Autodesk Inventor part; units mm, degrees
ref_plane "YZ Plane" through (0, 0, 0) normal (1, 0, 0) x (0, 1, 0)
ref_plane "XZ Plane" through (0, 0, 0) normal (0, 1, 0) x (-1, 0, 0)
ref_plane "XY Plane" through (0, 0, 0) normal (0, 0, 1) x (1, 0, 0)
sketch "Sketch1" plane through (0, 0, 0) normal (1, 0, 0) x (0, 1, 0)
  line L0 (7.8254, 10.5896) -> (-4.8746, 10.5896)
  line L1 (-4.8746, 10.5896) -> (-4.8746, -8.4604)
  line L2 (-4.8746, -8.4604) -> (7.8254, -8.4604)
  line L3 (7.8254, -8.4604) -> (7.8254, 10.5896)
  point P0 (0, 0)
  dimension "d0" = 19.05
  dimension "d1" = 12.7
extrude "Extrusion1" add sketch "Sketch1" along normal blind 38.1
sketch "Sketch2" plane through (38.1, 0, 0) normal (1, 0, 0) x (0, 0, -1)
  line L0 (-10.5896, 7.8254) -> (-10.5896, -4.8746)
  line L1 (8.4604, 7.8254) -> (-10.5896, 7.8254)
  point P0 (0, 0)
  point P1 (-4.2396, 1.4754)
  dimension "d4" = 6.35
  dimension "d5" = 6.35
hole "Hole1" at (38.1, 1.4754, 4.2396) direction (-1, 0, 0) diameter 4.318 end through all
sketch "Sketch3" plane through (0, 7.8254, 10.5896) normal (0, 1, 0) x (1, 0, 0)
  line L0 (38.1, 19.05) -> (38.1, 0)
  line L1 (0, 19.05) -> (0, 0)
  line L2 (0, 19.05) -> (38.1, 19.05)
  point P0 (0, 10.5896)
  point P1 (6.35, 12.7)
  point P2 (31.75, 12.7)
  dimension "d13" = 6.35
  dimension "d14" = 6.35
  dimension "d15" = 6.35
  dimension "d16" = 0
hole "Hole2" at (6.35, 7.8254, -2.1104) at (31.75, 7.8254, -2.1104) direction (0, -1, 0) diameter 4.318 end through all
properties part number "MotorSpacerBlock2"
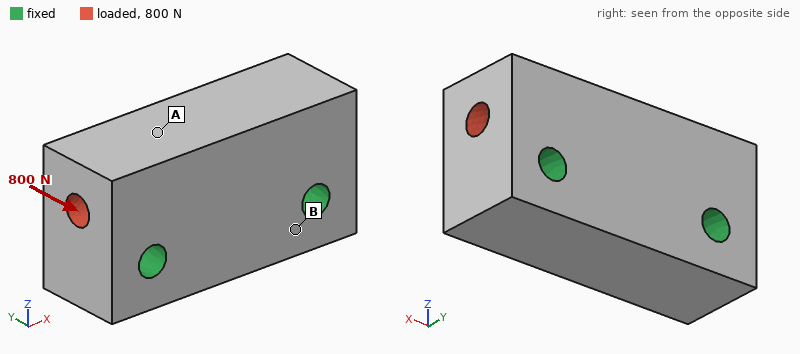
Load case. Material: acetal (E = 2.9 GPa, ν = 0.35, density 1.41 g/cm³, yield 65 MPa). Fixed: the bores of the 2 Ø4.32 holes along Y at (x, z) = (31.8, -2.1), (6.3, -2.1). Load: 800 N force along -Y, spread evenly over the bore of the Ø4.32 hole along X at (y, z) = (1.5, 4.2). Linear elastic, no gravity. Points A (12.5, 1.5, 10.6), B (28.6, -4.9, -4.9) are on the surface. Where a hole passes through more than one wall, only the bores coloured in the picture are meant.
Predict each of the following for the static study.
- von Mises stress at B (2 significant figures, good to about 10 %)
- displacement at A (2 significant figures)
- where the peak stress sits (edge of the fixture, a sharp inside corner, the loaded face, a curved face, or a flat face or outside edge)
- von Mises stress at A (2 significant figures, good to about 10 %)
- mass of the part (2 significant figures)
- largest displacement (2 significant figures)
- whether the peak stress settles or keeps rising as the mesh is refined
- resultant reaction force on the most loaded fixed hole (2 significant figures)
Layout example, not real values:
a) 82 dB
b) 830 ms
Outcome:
a) 3.3 MPa
b) 39 µm
c) edge of the fixture
d) 1.6 MPa
e) 12 g
f) 45 µm
g) keeps rising
h) 400 N
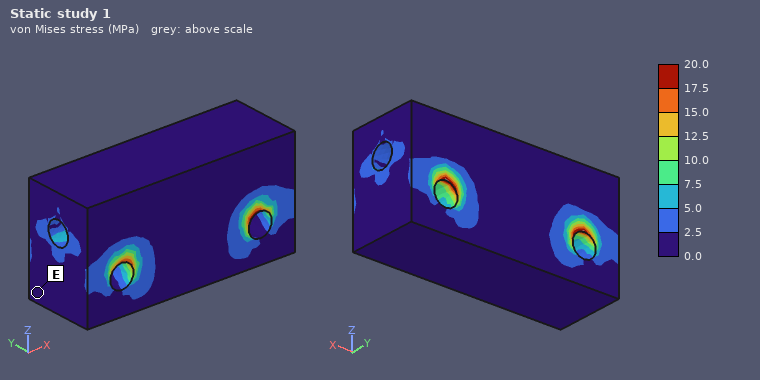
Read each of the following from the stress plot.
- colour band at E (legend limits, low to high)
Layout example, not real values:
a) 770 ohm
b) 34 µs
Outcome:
a) 0.0 to 2.5 MPa
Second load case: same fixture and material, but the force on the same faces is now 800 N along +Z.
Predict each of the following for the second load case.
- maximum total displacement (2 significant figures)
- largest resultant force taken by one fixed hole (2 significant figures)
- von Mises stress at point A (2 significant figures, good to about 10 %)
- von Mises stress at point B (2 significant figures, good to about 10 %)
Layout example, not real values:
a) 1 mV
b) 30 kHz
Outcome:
a) 15 µm
b) 400 N
c) 1.6 MPa
d) 2.0 MPa
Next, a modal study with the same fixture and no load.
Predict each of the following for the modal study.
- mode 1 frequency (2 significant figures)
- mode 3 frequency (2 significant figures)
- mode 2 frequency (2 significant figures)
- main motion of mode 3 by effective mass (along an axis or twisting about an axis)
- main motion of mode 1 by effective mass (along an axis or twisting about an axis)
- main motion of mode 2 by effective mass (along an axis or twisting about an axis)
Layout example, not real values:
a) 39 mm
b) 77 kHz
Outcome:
a) 8900 Hz
b) 13 kHz
c) 12 kHz
d) along Z
e) along Y
f) twisting about Z
